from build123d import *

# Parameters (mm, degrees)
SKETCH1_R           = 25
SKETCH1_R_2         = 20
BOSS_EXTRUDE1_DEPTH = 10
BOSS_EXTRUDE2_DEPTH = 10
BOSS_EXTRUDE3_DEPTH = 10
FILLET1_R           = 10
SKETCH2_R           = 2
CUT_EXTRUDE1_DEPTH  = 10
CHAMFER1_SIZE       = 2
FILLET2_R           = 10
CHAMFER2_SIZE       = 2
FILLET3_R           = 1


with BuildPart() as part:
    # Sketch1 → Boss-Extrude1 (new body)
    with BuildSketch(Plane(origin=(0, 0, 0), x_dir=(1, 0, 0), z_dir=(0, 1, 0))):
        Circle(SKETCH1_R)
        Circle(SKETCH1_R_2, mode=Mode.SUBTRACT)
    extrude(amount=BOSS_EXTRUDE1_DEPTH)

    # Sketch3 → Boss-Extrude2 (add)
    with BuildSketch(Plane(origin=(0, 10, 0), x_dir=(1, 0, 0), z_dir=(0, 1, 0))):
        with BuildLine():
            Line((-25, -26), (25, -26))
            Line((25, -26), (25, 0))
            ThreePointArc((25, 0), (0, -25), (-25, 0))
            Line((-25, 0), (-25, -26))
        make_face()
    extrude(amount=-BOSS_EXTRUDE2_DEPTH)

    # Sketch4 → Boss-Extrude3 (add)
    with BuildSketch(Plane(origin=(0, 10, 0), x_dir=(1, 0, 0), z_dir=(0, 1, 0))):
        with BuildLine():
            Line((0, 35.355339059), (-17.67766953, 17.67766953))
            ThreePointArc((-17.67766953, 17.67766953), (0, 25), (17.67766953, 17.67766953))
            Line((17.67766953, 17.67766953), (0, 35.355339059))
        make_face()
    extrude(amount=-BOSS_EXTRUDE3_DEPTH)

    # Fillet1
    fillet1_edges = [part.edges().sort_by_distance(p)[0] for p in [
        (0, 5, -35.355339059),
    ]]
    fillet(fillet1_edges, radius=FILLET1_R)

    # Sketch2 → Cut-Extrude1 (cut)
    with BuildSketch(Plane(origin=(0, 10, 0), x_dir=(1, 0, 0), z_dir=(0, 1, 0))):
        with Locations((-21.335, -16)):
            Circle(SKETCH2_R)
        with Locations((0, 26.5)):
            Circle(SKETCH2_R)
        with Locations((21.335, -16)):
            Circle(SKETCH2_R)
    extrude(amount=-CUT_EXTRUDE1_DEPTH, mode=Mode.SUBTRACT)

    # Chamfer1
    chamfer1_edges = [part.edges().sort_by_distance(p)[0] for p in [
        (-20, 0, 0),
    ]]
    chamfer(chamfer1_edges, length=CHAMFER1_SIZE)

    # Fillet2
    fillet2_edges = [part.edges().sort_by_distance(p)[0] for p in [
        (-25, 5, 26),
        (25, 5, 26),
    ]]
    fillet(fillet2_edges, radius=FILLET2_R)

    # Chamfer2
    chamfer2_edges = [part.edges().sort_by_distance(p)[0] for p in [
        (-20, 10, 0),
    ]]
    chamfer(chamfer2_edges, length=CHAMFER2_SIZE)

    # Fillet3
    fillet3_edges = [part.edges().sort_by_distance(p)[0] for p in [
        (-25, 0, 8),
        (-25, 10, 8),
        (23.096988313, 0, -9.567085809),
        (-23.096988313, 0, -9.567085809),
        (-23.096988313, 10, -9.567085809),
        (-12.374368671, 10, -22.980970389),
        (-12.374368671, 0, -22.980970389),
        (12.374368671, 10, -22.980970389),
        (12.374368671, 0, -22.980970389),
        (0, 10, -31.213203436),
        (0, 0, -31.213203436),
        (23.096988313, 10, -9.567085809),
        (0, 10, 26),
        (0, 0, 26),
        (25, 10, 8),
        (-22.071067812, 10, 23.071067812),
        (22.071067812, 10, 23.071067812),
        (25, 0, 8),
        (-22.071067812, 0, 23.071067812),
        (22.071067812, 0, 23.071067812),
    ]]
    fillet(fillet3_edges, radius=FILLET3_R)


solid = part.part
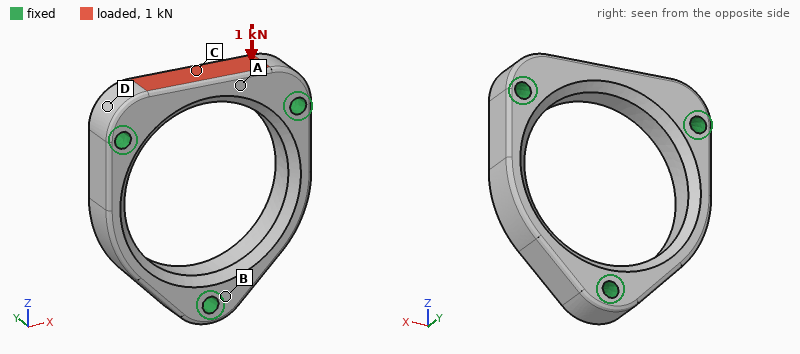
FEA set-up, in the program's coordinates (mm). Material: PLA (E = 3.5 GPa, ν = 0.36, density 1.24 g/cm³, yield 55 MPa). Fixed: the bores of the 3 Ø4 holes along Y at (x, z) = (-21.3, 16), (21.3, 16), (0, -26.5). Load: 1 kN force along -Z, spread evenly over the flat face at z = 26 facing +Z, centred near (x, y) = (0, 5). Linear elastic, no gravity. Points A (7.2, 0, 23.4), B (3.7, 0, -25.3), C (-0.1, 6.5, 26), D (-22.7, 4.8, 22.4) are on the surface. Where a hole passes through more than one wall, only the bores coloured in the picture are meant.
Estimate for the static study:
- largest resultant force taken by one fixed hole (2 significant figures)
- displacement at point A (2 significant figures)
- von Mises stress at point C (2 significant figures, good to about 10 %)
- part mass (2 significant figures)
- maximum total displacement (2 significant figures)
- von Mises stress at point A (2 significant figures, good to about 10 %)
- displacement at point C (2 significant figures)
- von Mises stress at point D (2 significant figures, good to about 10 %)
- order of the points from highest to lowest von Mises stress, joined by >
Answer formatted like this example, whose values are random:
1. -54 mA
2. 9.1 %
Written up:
1. 720 N
2. 0.11 mm
3. 22 MPa
4. 12 g
5. 0.16 mm
6. 10 MPa
7. 0.15 mm
8. 4.5 MPa
9. C > A > D > B
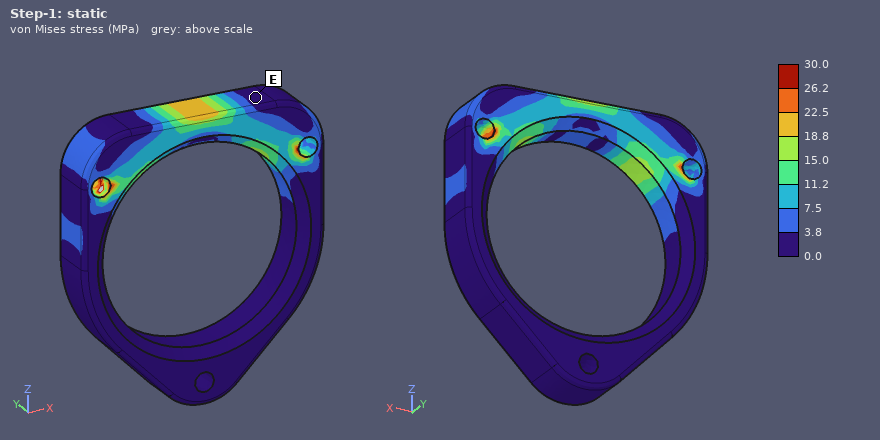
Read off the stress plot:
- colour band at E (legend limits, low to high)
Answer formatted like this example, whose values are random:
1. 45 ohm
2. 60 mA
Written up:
1. 0.0 to 3.8 MPa
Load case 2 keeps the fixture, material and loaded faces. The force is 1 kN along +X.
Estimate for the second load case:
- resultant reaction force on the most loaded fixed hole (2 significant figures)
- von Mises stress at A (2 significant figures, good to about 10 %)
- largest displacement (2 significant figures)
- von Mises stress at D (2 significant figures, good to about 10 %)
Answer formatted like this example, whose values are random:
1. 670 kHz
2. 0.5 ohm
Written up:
1. 530 N
2. 3.7 MPa
3. 46 µm
4. 3.0 MPa
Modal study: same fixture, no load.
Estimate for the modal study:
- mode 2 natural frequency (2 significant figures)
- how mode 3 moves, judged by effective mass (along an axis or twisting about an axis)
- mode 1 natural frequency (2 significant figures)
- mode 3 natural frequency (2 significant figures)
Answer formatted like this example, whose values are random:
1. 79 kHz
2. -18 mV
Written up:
1. 5500 Hz
2. along Y
3. 5400 Hz
4. 7300 Hz
